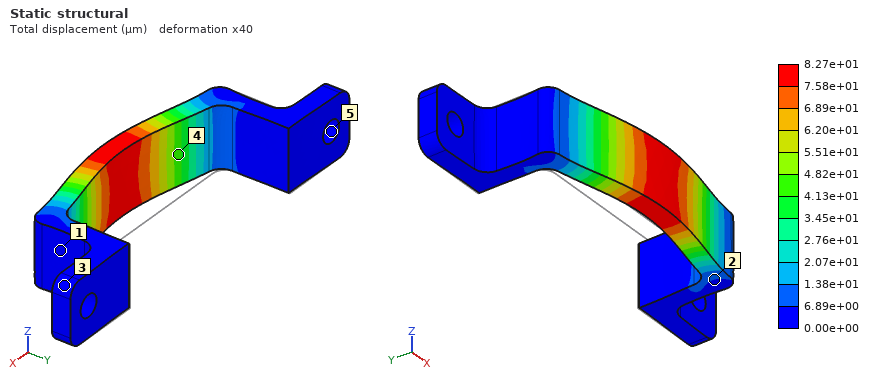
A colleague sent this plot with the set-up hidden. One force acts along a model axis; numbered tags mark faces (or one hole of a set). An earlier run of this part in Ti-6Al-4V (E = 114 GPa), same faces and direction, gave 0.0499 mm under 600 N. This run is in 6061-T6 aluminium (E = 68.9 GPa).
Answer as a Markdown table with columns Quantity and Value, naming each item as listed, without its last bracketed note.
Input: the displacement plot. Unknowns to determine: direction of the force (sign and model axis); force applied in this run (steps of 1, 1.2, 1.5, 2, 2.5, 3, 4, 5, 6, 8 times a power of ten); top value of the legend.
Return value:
| Quantity | Value |
|---|---|
| direction of the force | -Y |
| force applied in this run | 600 N |
| top value of the legend | 8.27e+01 µm |
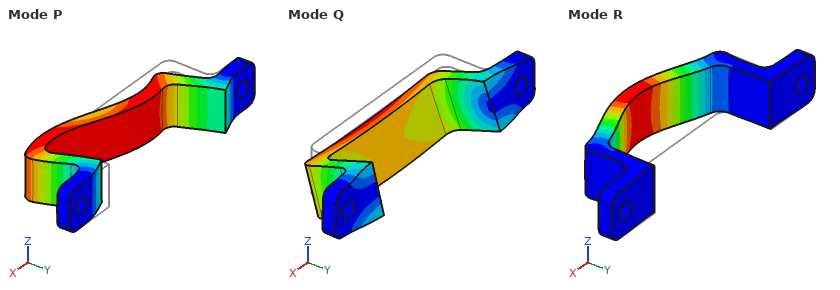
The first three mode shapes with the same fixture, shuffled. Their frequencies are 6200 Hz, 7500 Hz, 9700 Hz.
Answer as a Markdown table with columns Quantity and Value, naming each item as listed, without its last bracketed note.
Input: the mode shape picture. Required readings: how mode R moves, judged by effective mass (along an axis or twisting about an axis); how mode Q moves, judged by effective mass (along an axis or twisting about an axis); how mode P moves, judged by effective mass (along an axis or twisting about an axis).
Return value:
| Quantity | Value |
|---|---|
| how mode R moves, judged by effective mass | along Y |
| how mode Q moves, judged by effective mass | along Z |
| how mode P moves, judged by effective mass | along X |
